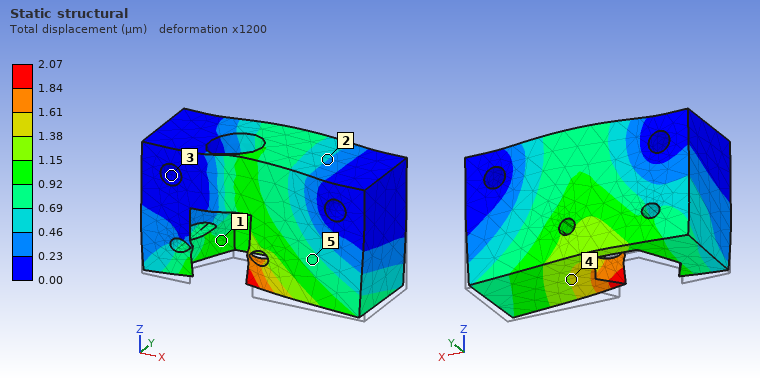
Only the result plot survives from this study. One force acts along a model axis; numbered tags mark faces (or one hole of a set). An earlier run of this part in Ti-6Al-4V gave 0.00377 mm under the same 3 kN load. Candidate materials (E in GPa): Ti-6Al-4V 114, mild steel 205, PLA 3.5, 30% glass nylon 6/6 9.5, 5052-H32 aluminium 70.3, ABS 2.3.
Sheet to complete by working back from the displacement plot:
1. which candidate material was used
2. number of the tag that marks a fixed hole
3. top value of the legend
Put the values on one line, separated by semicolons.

mild steel; 3; 2.07 µm
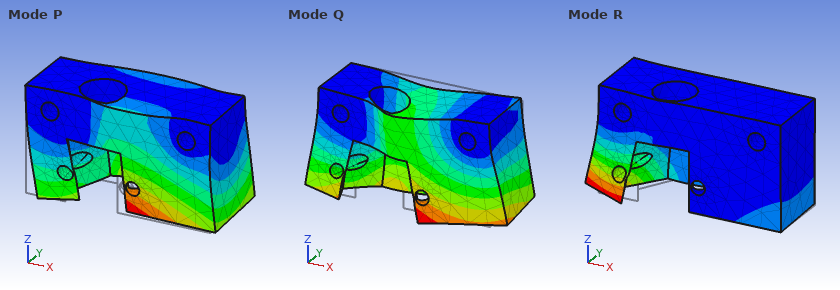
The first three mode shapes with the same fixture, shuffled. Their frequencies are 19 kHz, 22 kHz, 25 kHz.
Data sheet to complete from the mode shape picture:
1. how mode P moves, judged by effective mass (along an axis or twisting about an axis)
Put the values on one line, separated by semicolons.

along Y
